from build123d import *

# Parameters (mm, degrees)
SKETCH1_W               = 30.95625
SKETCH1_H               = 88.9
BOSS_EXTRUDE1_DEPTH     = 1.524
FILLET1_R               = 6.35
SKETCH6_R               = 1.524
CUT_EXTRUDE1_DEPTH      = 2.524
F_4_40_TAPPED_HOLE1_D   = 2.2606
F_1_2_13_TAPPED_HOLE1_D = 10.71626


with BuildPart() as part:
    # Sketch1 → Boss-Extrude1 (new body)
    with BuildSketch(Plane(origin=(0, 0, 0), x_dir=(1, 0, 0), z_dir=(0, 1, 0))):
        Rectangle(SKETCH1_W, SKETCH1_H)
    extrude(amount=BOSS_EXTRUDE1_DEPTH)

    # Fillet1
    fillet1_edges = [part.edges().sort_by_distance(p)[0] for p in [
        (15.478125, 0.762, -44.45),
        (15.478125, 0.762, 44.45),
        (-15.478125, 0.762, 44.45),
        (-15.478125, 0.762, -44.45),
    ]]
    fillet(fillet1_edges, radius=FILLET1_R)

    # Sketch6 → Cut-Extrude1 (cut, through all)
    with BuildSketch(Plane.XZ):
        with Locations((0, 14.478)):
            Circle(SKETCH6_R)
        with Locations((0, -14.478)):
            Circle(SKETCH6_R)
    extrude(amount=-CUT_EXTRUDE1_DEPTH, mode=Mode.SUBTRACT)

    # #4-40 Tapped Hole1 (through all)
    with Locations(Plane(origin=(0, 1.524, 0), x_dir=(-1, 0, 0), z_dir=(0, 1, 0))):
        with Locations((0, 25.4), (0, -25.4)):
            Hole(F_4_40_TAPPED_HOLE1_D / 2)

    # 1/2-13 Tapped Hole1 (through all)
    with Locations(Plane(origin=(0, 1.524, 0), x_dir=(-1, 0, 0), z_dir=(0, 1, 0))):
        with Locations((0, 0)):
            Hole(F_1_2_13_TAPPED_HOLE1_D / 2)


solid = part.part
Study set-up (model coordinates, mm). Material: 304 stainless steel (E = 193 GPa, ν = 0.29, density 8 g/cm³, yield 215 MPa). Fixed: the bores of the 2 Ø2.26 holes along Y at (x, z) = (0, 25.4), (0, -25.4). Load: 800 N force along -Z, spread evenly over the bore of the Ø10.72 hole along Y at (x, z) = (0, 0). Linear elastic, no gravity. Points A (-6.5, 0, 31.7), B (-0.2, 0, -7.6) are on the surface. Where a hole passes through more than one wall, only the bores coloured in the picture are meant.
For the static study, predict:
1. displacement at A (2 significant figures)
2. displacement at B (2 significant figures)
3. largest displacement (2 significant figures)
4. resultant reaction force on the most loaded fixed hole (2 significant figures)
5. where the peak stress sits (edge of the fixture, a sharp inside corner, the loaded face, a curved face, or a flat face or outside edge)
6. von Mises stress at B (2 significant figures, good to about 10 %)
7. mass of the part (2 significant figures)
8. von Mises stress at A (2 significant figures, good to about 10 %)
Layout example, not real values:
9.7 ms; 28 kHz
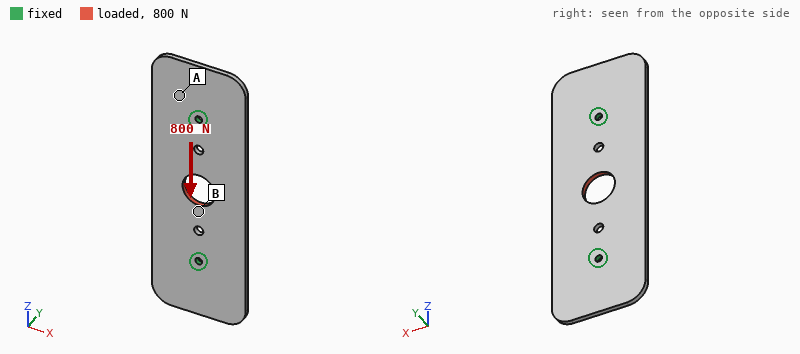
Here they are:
0.66 µm; 1.8 µm; 2.2 µm; 400 N; edge of the fixture; 16 MPa; 32 g; 5.2 MPa
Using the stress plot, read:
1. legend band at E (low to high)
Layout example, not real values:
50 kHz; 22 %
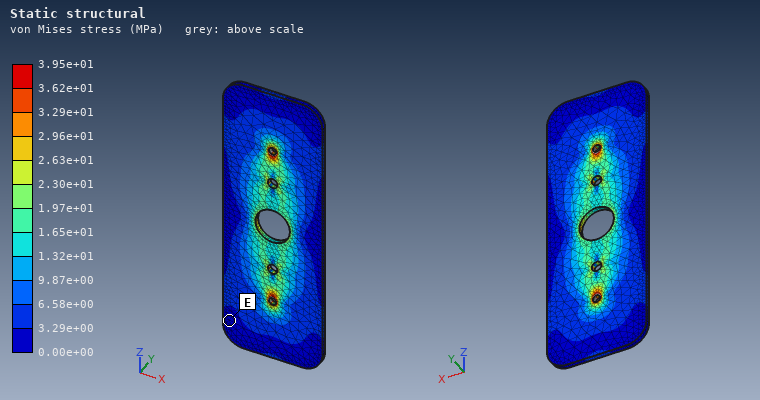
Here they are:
0.00e+00 to 3.29e+00 MPa
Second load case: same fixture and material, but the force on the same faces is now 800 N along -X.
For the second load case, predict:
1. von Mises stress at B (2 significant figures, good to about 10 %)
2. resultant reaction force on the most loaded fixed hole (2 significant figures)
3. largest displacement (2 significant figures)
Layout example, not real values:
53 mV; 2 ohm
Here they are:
24 MPa; 400 N; 6.5 µm
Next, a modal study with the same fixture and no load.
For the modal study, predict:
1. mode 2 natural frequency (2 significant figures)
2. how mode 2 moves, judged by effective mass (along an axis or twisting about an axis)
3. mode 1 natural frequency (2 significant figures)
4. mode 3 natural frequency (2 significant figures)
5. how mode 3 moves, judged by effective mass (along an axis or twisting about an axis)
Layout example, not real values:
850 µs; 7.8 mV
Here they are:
2500 Hz; twisting about Z; 2200 Hz; 2900 Hz; twisting about X
